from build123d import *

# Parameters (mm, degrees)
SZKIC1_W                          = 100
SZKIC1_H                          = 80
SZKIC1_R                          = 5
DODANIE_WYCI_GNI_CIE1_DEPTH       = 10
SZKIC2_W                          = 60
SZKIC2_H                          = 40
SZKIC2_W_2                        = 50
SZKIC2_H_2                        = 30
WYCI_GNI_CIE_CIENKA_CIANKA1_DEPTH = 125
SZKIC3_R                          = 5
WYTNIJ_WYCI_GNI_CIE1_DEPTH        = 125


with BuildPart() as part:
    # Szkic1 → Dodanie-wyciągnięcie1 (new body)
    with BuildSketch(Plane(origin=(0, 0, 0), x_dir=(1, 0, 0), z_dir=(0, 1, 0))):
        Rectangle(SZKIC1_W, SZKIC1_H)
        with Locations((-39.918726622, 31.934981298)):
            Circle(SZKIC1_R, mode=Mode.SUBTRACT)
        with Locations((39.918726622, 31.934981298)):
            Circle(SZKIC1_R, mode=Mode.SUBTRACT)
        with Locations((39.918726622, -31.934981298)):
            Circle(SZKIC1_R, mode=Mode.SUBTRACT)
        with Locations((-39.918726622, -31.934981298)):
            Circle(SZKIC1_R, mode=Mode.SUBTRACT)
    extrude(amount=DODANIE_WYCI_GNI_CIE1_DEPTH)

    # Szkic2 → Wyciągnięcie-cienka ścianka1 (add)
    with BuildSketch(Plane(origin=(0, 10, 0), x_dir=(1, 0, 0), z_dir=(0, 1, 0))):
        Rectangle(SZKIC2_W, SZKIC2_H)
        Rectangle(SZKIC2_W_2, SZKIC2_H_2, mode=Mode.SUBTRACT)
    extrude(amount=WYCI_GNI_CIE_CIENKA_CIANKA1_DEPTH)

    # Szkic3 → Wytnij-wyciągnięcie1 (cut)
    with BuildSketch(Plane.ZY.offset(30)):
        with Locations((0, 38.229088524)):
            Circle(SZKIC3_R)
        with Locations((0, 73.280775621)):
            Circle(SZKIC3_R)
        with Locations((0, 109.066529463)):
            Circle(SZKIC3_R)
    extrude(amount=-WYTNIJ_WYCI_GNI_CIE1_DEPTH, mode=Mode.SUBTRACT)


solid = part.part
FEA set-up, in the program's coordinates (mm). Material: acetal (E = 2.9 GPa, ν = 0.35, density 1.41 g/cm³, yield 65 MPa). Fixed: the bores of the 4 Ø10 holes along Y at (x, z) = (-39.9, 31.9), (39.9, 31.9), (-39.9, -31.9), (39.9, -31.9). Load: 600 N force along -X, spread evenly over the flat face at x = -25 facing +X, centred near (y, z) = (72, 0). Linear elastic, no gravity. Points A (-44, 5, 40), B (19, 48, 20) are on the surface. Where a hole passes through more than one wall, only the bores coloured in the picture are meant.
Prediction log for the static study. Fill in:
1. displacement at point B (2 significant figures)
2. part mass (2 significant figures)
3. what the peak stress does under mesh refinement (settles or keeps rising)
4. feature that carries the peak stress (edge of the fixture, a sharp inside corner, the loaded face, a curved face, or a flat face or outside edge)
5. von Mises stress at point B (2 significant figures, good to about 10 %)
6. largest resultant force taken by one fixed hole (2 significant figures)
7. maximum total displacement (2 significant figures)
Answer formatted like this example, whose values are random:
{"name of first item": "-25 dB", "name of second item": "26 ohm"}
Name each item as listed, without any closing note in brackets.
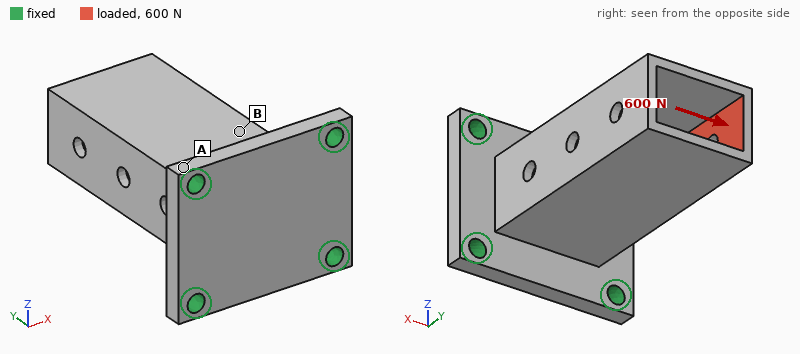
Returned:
{"displacement at point B": "0.14 mm", "part mass": "260 g", "what the peak stress does under mesh refinement": "keeps rising", "feature that carries the peak stress": "edge of the fixture", "von Mises stress at point B": "1.7 MPa", "largest resultant force taken by one fixed hole": "340 N", "maximum total displacement": "0.50 mm"}
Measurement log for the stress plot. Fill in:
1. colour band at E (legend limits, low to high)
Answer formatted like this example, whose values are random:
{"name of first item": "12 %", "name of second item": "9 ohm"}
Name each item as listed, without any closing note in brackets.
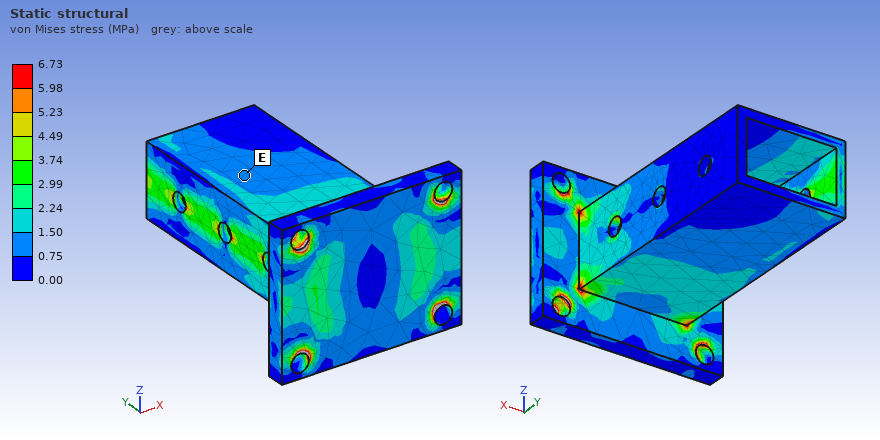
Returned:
{"colour band at E": "0.75 to 1.50 MPa"}
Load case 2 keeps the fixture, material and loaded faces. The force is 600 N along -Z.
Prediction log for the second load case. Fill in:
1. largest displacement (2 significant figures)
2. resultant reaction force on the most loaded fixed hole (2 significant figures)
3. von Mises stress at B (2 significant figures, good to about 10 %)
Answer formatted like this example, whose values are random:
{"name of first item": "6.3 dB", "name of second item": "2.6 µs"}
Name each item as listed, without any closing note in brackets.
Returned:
{"largest displacement": "0.96 mm", "resultant reaction force on the most loaded fixed hole": "500 N", "von Mises stress at B": "1.6 MPa"}
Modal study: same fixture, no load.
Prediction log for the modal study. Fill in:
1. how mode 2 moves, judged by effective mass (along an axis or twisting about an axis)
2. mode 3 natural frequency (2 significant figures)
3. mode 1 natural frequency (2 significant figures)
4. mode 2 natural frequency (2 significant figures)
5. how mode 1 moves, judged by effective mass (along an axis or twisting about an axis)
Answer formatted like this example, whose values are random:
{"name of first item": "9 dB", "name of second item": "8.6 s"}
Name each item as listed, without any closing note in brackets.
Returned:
{"how mode 2 moves, judged by effective mass": "along X", "mode 3 natural frequency": "1000 Hz", "mode 1 natural frequency": "420 Hz", "mode 2 natural frequency": "570 Hz", "how mode 1 moves, judged by effective mass": "along Z"}
